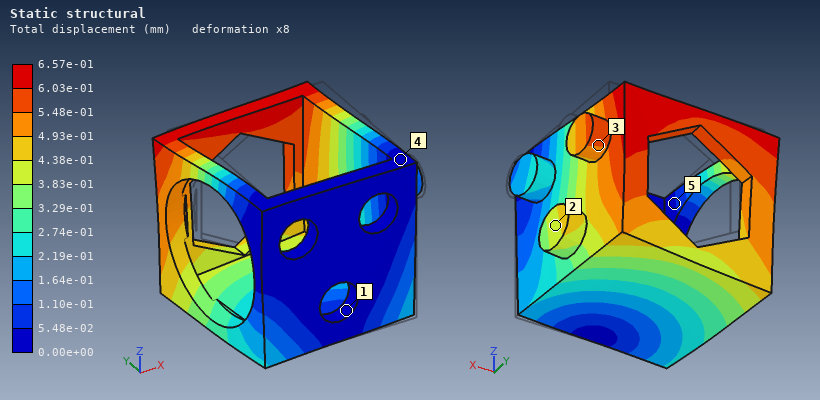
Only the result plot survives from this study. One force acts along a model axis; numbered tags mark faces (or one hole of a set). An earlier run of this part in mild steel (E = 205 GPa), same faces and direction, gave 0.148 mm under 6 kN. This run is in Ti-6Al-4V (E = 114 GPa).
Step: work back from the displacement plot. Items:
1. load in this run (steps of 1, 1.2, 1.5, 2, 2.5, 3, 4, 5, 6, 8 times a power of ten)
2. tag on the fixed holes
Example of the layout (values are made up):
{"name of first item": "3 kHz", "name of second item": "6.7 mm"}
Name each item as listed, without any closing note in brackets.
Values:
{"load in this run": "15 kN", "tag on the fixed holes": "1"}
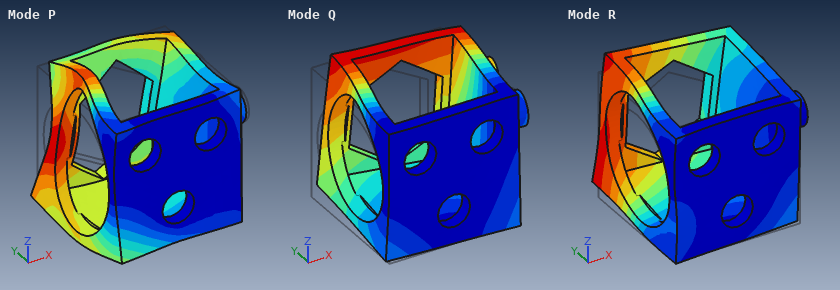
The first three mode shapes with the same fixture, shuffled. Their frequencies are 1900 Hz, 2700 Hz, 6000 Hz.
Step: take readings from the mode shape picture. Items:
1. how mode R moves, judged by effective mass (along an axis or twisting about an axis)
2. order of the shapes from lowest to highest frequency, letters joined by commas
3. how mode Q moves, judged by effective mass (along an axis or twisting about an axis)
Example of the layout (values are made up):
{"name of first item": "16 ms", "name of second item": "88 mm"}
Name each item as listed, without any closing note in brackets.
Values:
{"how mode R moves, judged by effective mass": "along Z", "order of the shapes from lowest to highest frequency, letters joined by commas": "Q, R, P", "how mode Q moves, judged by effective mass": "along X"}
